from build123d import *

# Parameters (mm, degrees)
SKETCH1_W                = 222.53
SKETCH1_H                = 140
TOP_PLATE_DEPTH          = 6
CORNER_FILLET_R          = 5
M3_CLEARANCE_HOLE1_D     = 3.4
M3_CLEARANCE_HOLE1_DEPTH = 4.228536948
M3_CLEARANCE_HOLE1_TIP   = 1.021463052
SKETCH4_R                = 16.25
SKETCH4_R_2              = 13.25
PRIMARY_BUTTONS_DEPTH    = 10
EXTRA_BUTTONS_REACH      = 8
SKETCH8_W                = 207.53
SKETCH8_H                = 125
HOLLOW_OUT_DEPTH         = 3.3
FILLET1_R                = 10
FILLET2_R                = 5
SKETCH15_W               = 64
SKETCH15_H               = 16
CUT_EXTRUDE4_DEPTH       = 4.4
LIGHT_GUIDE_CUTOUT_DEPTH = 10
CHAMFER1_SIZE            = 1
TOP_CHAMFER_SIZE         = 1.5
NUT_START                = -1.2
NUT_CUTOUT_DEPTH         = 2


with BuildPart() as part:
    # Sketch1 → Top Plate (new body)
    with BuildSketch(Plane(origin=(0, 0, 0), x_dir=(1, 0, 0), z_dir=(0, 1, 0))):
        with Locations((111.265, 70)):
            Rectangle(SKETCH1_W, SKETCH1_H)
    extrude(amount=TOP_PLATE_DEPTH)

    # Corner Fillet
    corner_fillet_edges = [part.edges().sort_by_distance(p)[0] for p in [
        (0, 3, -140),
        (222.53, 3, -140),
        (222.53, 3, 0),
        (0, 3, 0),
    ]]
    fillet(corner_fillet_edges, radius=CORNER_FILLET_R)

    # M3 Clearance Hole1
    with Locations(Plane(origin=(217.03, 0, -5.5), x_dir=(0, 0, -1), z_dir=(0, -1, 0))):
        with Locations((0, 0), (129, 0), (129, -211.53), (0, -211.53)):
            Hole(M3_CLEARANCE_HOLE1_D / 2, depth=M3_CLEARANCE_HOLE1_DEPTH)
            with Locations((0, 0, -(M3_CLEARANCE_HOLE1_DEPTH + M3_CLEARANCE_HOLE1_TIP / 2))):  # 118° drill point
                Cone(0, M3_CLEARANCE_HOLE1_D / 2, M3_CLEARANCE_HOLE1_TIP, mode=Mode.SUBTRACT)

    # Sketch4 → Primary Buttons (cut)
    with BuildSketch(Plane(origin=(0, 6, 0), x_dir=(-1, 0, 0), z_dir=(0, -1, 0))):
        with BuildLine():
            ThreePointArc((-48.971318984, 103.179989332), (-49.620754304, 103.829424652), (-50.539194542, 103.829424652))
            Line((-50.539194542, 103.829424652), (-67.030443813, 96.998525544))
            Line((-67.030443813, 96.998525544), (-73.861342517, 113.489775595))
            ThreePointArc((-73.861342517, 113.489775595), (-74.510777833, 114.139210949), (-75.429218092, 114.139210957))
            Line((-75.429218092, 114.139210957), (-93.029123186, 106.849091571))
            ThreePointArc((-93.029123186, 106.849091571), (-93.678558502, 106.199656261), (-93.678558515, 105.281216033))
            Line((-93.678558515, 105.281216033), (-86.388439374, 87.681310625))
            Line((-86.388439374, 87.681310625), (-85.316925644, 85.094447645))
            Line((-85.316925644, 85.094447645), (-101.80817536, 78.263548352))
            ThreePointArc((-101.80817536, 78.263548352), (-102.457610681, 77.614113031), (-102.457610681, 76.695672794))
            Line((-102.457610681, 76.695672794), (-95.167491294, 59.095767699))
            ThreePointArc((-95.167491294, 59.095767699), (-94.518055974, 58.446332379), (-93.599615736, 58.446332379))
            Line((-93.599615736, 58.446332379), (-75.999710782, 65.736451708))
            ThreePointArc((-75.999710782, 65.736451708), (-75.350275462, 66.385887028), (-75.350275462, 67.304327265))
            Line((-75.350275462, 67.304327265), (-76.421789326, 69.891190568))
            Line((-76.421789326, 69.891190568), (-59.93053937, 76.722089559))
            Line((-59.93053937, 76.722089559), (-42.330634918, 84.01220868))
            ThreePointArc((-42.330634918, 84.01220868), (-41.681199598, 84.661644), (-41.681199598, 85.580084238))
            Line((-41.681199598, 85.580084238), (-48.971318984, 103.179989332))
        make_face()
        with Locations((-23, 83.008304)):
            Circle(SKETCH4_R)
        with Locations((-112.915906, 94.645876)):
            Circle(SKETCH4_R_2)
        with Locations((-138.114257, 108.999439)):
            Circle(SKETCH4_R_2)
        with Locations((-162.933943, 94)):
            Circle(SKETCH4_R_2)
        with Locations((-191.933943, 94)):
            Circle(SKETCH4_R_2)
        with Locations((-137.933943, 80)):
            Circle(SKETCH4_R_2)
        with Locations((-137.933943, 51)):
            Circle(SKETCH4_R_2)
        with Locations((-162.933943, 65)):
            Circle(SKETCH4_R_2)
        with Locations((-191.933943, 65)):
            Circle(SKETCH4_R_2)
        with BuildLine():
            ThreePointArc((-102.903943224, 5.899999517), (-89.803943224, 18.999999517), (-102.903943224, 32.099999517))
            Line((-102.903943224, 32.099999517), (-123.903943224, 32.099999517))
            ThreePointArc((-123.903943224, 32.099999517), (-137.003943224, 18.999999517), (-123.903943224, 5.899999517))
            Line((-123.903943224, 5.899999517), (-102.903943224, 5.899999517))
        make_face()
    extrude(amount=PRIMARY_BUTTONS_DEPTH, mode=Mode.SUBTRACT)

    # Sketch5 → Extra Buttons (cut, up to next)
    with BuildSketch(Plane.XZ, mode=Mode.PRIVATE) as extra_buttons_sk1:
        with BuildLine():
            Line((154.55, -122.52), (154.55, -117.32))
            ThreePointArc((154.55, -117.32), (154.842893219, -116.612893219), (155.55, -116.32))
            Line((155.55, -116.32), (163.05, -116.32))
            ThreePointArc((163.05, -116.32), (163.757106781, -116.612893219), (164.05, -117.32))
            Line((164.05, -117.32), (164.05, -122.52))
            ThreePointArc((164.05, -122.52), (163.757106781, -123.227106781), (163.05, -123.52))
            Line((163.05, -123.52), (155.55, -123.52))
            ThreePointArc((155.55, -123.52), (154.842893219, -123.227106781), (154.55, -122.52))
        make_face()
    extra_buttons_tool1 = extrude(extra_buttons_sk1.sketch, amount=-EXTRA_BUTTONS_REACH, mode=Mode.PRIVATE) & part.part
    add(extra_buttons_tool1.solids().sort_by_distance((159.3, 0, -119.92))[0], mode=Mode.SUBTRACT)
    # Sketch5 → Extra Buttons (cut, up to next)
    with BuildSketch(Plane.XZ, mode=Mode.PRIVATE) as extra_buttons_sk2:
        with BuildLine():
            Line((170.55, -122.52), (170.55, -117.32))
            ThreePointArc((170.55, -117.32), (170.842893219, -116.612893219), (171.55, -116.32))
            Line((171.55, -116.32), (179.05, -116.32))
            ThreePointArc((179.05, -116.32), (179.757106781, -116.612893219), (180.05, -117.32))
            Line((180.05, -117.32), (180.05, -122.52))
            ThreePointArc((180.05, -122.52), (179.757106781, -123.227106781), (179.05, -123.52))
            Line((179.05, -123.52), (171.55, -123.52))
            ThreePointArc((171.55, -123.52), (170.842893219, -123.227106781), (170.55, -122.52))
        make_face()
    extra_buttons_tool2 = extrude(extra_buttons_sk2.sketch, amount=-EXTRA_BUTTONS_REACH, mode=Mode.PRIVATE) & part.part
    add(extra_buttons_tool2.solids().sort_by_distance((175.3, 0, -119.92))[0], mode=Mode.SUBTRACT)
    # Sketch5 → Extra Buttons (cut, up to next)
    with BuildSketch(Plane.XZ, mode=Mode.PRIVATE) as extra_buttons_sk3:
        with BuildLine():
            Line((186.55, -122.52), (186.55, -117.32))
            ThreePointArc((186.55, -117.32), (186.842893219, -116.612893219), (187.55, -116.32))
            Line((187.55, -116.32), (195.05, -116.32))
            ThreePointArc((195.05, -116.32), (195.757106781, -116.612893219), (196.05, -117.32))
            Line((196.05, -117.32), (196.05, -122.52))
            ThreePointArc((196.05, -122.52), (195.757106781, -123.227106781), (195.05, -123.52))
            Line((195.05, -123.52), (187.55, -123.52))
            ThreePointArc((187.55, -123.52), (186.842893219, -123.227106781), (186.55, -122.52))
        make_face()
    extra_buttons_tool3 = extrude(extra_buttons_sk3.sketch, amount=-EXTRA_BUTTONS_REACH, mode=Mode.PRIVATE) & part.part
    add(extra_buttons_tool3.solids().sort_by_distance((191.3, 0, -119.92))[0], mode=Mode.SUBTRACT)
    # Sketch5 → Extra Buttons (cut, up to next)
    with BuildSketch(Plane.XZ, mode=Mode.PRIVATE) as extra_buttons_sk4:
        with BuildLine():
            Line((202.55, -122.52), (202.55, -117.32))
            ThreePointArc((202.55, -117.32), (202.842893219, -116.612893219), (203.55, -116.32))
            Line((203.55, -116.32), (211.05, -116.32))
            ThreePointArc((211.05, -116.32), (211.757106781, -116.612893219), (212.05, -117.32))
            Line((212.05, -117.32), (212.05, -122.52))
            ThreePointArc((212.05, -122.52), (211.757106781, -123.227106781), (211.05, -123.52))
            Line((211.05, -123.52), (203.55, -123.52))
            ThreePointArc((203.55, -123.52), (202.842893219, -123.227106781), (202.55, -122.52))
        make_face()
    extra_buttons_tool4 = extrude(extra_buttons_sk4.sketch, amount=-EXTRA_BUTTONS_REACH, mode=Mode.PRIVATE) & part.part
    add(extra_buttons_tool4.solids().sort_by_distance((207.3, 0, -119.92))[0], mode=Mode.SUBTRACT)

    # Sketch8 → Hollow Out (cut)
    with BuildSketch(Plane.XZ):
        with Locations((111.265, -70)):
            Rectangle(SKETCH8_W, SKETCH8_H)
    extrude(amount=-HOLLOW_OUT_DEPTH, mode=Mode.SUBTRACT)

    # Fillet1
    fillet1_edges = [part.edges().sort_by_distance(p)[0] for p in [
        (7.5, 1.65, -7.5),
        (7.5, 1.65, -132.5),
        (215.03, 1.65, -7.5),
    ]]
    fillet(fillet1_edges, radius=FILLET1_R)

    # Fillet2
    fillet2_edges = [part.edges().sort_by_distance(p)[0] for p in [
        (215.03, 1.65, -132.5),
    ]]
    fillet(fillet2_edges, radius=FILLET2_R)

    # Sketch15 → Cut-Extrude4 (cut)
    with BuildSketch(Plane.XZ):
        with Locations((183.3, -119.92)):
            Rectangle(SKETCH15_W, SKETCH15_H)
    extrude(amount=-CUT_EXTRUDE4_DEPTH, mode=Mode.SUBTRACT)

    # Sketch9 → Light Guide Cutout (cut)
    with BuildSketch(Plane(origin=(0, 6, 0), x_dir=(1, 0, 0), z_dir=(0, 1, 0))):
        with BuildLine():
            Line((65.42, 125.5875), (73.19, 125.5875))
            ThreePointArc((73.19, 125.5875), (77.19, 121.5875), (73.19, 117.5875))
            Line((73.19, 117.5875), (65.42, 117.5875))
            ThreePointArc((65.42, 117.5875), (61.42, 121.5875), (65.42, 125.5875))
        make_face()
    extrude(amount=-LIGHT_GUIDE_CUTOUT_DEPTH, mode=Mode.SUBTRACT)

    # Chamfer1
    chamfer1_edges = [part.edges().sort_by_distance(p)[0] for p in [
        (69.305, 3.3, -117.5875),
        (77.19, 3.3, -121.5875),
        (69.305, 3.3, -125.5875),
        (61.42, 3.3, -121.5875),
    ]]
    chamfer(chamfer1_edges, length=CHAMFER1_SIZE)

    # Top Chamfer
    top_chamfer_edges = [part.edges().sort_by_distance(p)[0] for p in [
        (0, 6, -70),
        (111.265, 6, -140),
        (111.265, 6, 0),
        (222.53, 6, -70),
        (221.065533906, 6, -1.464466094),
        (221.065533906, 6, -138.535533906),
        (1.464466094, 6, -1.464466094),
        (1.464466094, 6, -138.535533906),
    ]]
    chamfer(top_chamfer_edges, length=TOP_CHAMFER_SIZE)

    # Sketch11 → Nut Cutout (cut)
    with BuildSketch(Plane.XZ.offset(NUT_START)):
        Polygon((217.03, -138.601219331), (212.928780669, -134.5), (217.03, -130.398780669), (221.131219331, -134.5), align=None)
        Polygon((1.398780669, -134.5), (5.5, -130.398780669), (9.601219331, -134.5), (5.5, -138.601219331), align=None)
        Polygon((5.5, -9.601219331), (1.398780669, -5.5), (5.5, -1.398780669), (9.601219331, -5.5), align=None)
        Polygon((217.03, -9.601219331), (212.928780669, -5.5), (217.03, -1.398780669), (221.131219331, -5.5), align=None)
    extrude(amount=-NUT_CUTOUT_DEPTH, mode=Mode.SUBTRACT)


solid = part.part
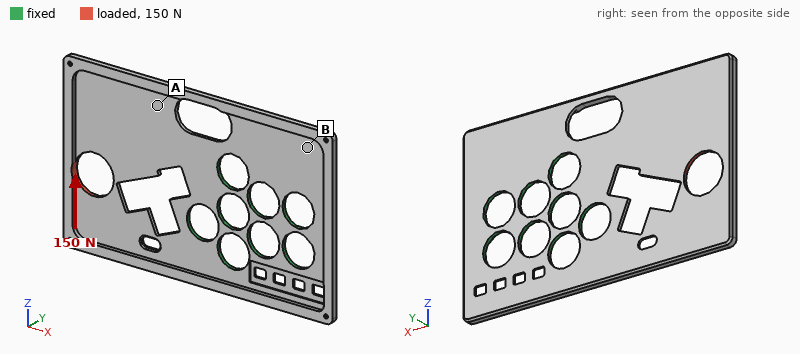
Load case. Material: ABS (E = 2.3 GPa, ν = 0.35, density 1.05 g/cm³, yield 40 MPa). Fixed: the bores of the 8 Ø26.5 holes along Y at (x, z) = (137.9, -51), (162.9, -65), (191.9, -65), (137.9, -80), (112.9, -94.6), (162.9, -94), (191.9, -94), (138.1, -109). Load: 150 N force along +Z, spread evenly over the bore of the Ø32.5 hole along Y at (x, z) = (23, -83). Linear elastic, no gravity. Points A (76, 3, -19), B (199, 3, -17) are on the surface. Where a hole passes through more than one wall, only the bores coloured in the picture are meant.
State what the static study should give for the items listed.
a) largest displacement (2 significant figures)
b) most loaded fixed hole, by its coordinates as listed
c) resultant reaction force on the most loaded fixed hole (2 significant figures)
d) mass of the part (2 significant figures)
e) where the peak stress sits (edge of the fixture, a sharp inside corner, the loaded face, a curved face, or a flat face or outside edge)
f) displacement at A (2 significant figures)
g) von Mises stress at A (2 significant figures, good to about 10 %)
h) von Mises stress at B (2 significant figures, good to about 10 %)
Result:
1.3 mm
(112.9, -94.6)
170 N
80 g
a curved face
0.35 mm
1.5 MPa
0.50 MPa
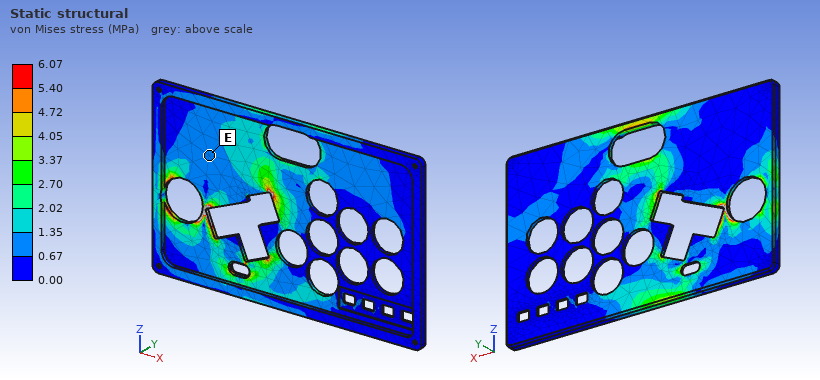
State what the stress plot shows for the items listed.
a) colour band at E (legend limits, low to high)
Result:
0.67 to 1.35 MPa
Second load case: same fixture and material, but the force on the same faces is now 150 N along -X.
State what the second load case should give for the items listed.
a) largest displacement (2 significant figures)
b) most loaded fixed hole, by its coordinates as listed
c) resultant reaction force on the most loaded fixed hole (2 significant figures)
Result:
0.19 mm
(137.9, -51)
79 N
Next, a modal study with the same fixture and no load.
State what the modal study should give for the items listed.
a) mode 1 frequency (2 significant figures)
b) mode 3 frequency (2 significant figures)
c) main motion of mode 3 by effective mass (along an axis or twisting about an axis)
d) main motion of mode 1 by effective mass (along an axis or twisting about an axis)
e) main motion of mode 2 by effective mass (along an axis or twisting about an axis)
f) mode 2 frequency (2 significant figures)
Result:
47 Hz
250 Hz
along Y
along Y
twisting about X
93 Hz
